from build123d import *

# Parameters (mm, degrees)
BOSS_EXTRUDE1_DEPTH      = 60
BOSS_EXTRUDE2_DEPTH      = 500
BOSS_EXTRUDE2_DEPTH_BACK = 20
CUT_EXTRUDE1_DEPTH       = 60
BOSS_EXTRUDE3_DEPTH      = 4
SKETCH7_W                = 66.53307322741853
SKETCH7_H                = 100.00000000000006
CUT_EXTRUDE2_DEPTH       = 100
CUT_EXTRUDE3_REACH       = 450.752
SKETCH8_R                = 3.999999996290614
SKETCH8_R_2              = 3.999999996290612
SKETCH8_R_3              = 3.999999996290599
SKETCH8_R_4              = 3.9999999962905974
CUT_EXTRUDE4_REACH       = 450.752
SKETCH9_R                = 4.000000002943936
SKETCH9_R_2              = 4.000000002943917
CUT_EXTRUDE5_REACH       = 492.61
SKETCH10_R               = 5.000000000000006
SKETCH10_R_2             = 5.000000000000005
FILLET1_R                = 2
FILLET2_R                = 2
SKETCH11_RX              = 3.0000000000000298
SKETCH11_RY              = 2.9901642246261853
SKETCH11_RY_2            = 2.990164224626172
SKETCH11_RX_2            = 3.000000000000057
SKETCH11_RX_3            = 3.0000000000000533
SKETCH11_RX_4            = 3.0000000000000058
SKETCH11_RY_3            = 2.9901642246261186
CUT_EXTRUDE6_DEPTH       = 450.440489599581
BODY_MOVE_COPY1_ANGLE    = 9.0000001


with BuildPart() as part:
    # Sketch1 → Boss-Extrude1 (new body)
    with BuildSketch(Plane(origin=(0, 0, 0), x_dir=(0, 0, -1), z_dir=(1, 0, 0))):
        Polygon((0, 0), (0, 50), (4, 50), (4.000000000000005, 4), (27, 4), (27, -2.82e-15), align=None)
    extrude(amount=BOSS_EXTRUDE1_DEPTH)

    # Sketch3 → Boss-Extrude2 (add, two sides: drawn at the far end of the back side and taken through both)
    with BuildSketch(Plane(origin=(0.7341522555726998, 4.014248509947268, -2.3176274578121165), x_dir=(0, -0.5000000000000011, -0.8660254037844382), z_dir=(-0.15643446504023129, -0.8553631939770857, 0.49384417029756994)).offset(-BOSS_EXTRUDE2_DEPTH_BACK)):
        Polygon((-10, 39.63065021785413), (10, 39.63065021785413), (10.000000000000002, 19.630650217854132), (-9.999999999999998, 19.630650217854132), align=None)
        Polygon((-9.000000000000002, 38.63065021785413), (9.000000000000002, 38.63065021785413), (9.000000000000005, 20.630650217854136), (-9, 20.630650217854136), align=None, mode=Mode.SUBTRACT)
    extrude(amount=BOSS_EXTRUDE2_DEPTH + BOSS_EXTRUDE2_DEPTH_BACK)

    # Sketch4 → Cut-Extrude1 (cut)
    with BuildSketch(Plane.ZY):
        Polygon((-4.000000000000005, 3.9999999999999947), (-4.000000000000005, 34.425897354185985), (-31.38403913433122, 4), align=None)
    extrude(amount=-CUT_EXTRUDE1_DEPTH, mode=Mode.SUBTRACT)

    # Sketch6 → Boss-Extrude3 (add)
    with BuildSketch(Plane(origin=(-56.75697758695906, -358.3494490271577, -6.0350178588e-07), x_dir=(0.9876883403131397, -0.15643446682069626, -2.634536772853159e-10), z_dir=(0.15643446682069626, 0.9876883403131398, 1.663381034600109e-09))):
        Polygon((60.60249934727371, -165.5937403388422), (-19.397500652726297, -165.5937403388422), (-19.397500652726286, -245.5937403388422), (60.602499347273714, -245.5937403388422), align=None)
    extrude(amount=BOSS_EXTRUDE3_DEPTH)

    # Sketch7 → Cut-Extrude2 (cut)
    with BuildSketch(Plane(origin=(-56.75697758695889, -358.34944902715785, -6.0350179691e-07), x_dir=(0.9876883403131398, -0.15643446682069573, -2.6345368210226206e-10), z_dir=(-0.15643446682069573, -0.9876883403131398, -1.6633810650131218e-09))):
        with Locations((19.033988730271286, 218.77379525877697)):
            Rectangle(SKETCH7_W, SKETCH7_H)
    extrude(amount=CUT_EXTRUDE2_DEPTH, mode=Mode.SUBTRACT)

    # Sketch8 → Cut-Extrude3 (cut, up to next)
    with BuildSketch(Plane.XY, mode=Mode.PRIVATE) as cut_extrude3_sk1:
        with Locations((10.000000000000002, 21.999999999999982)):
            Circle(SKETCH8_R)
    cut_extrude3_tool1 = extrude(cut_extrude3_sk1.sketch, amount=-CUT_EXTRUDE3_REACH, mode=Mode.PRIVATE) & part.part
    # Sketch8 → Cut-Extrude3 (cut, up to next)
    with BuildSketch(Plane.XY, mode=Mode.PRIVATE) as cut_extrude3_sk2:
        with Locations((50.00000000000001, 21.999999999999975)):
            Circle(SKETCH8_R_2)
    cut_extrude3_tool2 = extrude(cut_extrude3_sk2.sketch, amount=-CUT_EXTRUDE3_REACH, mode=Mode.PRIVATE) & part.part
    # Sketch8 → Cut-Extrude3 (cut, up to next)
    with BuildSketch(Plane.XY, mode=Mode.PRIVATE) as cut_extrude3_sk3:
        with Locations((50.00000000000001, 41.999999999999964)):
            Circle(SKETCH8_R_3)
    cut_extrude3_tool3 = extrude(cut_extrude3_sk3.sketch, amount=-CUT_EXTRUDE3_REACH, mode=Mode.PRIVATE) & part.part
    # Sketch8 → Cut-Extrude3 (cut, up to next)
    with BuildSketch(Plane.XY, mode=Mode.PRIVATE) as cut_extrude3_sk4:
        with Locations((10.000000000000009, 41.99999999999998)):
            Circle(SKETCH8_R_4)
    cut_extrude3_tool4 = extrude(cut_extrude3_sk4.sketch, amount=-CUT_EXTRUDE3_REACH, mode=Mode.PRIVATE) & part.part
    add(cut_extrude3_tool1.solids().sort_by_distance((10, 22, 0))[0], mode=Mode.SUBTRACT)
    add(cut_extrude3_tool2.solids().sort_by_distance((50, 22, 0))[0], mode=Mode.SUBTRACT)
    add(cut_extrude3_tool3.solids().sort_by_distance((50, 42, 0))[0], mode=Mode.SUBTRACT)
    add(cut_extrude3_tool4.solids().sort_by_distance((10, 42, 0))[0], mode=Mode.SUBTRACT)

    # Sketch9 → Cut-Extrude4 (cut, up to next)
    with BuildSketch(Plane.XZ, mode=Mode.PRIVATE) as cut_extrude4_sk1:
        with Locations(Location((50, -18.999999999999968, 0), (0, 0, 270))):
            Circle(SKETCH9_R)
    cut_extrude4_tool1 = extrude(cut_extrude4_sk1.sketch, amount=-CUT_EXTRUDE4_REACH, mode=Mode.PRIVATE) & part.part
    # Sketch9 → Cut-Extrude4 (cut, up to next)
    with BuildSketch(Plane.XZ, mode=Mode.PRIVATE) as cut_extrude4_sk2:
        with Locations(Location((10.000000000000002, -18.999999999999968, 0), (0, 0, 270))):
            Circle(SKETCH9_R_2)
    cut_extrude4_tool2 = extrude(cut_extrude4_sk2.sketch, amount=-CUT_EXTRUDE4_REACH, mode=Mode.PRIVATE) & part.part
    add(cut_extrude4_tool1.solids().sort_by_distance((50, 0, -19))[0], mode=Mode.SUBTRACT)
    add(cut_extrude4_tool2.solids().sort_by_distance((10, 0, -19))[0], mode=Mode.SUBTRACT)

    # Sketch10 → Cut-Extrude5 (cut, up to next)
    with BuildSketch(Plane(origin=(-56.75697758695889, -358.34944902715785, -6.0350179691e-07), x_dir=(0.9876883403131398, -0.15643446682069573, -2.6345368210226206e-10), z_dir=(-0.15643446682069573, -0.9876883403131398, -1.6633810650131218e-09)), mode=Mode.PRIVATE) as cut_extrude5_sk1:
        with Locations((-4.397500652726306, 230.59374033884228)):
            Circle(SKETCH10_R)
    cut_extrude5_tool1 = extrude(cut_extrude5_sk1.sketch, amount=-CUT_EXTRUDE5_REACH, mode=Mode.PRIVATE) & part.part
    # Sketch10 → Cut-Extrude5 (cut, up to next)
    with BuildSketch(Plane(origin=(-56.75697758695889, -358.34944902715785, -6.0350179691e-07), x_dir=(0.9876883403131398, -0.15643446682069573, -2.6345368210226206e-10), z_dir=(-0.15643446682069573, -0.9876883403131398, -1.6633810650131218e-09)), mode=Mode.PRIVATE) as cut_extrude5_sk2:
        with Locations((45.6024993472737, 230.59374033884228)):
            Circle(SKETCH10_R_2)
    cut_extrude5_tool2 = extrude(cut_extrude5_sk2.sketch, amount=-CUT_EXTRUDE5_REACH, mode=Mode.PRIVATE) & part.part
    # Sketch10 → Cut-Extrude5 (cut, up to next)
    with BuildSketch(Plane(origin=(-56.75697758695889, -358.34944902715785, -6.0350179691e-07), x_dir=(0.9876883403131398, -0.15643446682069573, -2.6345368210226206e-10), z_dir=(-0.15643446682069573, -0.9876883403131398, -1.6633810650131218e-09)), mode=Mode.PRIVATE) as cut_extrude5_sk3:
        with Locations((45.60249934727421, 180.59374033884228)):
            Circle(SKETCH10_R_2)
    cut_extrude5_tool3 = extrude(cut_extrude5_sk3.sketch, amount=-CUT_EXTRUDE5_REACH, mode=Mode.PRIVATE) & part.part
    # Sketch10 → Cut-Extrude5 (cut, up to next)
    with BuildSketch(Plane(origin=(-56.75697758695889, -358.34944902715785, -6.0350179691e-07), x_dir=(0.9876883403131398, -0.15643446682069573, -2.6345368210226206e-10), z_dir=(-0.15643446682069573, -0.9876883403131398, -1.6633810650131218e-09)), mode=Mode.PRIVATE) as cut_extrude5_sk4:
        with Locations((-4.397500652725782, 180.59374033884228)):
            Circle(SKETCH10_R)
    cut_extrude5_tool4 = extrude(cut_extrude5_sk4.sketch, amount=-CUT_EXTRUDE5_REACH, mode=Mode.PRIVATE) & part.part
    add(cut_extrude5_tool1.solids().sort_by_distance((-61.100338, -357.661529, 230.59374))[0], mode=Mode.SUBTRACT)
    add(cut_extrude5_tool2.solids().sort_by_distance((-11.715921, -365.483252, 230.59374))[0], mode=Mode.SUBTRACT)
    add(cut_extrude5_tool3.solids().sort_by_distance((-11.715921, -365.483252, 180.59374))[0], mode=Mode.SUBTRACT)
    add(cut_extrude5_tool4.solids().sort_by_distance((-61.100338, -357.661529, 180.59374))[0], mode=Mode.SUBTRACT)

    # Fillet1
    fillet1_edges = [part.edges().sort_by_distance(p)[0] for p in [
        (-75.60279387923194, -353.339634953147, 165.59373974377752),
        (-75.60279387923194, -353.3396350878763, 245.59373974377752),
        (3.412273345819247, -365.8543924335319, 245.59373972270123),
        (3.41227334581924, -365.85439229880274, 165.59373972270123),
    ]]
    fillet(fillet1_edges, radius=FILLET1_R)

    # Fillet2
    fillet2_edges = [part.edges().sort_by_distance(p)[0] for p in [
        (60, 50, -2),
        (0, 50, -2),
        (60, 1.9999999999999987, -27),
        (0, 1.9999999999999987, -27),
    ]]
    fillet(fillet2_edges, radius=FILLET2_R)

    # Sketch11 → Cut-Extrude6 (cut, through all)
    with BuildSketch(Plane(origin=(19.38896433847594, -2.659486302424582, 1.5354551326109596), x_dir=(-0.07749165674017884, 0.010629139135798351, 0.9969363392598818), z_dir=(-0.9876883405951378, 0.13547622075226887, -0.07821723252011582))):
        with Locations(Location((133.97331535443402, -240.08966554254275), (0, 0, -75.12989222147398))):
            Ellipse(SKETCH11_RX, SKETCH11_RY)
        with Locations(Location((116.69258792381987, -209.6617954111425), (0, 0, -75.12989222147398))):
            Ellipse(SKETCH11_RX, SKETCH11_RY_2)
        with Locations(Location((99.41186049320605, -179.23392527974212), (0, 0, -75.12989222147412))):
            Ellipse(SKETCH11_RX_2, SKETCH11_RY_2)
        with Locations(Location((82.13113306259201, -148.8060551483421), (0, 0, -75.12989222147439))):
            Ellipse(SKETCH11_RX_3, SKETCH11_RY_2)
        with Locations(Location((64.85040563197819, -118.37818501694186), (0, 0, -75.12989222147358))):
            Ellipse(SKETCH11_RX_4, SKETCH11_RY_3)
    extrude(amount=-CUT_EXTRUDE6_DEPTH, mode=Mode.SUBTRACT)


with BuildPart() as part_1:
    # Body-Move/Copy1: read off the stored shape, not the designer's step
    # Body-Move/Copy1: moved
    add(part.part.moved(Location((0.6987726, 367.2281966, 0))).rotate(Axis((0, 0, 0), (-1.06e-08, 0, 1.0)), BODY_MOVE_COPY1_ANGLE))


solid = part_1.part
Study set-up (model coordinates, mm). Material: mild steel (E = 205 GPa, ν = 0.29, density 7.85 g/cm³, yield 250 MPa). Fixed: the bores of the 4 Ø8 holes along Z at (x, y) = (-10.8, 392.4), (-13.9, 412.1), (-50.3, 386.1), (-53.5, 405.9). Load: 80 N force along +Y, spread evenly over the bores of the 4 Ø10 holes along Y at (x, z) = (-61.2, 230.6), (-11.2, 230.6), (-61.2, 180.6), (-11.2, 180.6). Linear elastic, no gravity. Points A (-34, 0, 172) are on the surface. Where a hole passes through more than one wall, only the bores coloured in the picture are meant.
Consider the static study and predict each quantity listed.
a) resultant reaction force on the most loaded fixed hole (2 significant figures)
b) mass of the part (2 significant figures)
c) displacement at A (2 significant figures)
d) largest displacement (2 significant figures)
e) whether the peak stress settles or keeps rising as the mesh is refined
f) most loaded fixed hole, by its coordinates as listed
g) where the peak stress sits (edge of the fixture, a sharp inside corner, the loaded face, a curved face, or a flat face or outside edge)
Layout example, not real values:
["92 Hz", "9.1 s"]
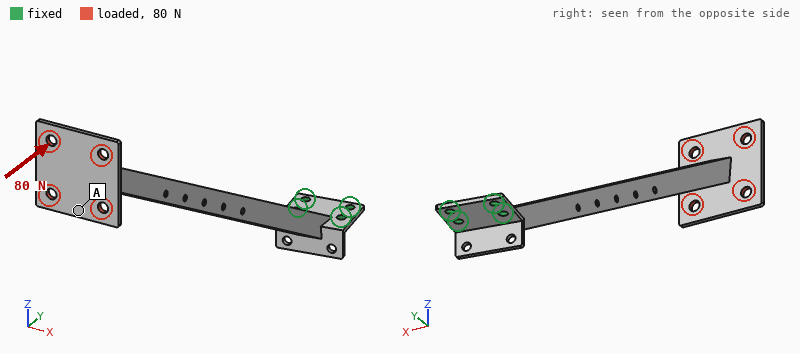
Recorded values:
["170 N", "570 g", "2.0 mm", "2.2 mm", "keeps rising", "(-50.3, 386.1)", "edge of the fixture"]
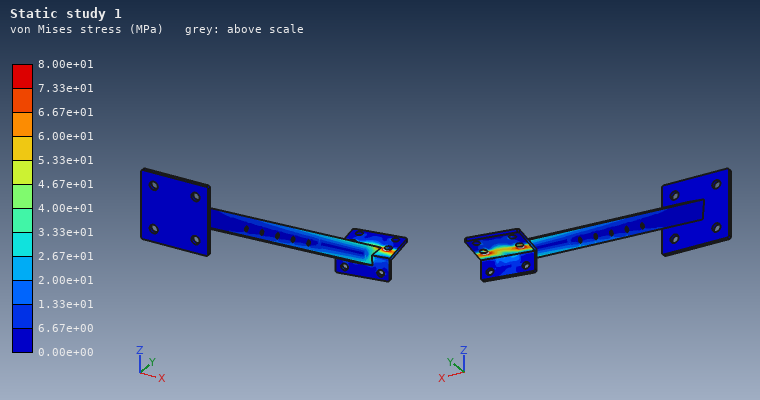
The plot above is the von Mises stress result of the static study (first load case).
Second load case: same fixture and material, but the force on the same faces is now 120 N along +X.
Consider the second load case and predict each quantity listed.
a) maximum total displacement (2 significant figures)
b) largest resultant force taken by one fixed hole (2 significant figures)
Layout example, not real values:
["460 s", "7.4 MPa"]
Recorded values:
["4.0 mm", "1.3 kN"]
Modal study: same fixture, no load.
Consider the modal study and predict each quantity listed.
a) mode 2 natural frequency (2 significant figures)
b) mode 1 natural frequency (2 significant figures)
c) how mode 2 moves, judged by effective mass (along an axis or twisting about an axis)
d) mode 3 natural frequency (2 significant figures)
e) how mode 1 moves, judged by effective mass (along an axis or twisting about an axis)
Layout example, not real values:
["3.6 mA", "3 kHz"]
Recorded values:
["57 Hz", "43 Hz", "along X", "410 Hz", "along Z"]
